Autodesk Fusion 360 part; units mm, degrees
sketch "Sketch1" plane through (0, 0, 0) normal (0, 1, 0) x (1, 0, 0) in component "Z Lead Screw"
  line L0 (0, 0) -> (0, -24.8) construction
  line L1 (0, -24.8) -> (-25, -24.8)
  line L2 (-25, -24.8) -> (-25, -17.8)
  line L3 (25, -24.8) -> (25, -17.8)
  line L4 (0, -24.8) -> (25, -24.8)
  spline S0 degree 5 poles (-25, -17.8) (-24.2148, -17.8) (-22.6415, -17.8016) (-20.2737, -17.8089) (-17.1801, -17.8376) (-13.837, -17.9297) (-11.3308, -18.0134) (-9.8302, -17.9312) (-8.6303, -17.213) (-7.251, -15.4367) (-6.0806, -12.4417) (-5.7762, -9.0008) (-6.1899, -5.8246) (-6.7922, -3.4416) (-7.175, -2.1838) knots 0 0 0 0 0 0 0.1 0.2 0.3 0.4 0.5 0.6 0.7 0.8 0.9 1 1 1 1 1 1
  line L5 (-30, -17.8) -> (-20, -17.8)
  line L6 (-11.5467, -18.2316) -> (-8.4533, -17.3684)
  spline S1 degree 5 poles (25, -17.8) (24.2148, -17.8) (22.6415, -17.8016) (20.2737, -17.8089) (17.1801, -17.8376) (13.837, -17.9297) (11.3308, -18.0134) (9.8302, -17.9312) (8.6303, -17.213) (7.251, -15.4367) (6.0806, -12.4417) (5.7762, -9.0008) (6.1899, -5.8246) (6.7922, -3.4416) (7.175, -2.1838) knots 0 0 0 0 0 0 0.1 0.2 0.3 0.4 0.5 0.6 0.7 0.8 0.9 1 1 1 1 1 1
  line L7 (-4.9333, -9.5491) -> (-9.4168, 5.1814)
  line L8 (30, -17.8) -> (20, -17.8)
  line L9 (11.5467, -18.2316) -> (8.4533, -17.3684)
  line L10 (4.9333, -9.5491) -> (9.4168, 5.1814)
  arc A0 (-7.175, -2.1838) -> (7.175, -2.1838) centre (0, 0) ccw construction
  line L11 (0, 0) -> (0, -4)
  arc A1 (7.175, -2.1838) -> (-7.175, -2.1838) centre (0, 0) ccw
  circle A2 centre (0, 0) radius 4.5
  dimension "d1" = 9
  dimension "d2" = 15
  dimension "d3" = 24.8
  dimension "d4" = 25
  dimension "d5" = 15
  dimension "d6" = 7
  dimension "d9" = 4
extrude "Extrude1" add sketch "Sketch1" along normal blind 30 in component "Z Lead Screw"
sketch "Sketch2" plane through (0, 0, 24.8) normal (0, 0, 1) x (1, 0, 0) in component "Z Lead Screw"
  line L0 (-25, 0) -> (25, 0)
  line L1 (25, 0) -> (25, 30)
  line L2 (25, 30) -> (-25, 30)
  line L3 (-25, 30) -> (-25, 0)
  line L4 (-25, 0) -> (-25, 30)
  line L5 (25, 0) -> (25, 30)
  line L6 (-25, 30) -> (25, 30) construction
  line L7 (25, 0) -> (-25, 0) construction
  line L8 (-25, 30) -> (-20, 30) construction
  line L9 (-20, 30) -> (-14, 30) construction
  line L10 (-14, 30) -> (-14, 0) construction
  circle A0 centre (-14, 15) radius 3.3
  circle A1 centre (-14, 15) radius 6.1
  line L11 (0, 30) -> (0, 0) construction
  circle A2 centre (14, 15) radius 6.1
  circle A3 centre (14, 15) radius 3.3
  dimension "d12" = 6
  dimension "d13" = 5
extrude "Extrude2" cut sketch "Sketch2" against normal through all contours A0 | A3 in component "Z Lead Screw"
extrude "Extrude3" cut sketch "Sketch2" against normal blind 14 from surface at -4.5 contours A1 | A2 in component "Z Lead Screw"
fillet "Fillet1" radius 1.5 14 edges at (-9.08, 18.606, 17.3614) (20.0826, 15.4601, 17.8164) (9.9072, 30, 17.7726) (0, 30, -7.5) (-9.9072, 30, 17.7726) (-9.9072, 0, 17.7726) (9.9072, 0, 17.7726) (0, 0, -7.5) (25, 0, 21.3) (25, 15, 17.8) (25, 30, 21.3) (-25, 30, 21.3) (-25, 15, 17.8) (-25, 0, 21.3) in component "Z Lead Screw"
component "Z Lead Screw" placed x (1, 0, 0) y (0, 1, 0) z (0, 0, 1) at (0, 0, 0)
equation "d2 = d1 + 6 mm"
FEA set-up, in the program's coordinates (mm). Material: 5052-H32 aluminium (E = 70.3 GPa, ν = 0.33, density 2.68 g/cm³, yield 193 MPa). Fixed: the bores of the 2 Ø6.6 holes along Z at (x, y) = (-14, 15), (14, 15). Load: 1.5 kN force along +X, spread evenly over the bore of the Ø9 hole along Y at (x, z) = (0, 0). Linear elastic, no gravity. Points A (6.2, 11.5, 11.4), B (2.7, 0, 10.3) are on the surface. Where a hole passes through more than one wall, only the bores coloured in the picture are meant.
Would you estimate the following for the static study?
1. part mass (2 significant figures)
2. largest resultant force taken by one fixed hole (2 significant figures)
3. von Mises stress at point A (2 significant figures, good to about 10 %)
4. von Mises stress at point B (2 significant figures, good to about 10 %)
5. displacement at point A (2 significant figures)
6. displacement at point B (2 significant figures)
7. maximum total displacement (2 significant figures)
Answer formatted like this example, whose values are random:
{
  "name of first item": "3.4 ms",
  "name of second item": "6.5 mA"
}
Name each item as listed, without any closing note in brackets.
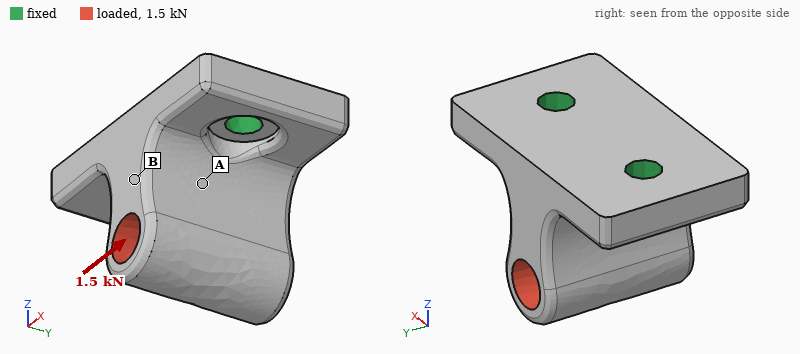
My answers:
{
  "part mass": "47 g",
  "largest resultant force taken by one fixed hole": "1.6 kN",
  "von Mises stress at point A": "28 MPa",
  "von Mises stress at point B": "8.8 MPa",
  "displacement at point A": "9.0 µm",
  "displacement at point B": "7.8 µm",
  "maximum total displacement": "37 µm"
}
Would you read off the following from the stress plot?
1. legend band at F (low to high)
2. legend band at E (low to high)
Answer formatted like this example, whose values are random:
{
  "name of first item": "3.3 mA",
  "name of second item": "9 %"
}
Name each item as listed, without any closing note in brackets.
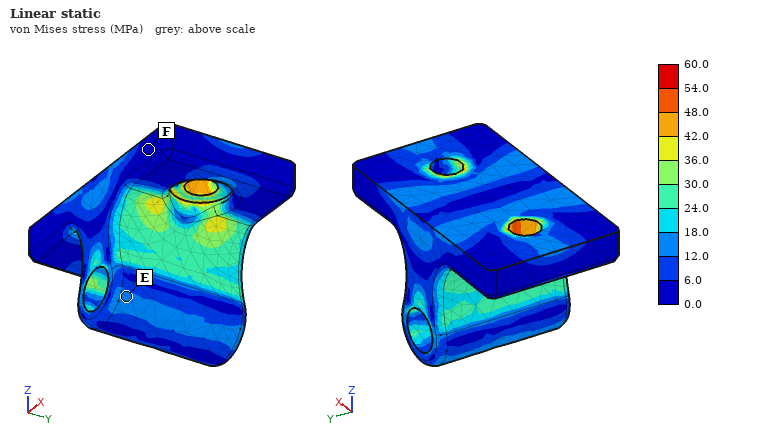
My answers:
{
  "legend band at F": "0.0 to 6.0 MPa",
  "legend band at E": "12.0 to 18.0 MPa"
}
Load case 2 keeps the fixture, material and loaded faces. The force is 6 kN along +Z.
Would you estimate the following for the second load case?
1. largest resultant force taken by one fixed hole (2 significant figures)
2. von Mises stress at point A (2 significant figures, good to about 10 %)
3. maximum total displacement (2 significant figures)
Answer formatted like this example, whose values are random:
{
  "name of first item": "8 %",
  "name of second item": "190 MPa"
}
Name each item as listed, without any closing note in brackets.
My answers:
{
  "largest resultant force taken by one fixed hole": "3.3 kN",
  "von Mises stress at point A": "33 MPa",
  "maximum total displacement": "25 µm"
}
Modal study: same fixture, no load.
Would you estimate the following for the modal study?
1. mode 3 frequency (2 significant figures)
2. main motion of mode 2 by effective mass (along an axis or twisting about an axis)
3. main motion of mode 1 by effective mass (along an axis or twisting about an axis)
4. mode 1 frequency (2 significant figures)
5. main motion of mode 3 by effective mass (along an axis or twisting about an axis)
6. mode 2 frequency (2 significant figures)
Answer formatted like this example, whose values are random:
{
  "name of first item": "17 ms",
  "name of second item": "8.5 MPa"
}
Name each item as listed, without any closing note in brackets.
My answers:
{
  "mode 3 frequency": "18 kHz",
  "main motion of mode 2 by effective mass": "along X",
  "main motion of mode 1 by effective mass": "along Y",
  "mode 1 frequency": "6100 Hz",
  "main motion of mode 3 by effective mass": "along Z",
  "mode 2 frequency": "11 kHz"
}
